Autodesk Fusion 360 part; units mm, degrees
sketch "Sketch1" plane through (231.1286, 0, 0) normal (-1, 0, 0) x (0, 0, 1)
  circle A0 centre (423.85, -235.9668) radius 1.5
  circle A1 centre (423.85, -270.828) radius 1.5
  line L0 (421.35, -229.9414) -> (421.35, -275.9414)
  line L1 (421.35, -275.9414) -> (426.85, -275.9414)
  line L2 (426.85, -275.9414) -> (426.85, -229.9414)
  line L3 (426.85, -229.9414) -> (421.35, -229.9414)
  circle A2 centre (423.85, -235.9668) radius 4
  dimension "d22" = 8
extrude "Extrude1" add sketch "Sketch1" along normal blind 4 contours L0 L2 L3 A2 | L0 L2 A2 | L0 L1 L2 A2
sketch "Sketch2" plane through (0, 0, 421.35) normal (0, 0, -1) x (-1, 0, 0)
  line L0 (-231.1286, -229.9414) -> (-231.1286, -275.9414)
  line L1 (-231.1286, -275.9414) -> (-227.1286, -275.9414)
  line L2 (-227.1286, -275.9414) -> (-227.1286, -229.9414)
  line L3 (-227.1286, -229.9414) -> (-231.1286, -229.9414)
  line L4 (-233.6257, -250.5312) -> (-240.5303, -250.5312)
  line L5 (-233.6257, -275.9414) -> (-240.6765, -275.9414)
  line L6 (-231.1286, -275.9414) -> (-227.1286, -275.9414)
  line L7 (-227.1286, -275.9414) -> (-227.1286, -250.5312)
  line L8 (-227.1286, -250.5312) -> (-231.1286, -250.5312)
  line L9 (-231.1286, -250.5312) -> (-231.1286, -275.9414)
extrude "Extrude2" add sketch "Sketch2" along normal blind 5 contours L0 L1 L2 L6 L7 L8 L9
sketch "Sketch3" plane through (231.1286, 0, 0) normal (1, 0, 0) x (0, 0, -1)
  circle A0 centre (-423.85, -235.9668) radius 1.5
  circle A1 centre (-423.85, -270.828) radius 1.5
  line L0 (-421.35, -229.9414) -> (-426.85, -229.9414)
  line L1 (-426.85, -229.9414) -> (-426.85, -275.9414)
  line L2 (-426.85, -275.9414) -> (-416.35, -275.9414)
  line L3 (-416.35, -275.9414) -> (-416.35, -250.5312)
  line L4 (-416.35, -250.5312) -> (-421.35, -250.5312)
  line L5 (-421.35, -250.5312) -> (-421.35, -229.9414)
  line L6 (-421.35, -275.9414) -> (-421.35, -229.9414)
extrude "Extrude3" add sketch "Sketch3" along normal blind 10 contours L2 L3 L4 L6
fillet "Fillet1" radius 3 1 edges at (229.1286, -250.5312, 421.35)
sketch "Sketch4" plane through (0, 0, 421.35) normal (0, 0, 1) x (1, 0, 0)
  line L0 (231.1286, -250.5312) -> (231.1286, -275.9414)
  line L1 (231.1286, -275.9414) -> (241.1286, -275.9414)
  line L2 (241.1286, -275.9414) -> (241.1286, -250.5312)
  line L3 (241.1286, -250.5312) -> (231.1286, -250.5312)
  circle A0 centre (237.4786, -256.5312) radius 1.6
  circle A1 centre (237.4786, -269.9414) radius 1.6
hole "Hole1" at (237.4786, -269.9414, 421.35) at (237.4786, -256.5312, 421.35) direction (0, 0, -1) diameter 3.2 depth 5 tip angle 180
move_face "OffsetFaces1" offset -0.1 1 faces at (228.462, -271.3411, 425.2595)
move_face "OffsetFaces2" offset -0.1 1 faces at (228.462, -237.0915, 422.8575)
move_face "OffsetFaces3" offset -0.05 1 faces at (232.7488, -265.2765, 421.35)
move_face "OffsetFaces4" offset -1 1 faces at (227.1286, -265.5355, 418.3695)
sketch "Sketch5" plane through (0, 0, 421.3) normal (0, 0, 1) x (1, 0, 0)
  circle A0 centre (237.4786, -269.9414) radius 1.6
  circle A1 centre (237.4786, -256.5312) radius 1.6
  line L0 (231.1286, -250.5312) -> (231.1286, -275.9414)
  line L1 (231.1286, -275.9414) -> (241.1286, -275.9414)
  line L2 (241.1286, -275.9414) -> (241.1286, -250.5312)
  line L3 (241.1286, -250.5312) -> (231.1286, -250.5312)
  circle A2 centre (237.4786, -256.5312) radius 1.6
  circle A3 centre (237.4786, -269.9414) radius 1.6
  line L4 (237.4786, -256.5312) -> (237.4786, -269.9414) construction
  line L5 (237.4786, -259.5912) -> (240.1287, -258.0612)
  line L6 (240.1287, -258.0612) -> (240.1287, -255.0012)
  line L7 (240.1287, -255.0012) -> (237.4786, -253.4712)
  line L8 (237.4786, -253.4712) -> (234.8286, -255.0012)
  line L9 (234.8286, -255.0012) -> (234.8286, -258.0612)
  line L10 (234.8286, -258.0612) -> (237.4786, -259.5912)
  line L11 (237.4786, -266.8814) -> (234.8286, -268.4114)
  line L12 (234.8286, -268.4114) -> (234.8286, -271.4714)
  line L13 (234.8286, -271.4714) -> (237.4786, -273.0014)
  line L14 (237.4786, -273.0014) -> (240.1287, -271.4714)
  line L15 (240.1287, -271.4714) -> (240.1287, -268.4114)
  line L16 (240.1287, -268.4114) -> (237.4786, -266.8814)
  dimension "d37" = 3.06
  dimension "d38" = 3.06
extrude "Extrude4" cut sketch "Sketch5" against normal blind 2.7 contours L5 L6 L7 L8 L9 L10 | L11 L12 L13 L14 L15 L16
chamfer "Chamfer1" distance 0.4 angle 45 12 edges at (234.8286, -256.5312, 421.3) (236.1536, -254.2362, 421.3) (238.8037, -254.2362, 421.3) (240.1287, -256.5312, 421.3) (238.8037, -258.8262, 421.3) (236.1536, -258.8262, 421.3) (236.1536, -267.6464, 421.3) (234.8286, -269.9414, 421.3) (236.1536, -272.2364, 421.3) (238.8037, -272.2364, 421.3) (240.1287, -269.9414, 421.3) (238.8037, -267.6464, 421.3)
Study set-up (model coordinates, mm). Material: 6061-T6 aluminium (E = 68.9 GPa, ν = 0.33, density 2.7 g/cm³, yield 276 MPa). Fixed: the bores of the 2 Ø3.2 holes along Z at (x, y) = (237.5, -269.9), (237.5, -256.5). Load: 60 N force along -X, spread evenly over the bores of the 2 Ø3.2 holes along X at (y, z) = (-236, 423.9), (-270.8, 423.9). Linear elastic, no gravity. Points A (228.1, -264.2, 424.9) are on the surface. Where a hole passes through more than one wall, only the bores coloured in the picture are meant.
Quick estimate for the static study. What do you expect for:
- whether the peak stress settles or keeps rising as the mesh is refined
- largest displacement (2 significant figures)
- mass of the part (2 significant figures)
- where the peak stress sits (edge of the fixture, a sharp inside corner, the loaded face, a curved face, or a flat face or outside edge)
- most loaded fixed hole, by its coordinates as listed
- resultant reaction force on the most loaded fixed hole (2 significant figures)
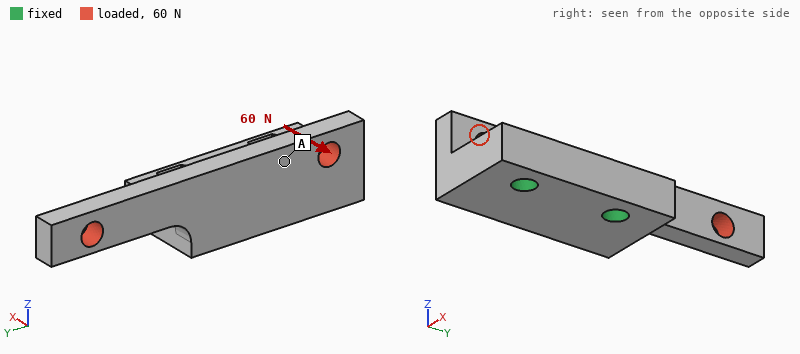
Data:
keeps rising
99 µm
5.9 g
a sharp inside corner
(237.5, -256.5)
69 N
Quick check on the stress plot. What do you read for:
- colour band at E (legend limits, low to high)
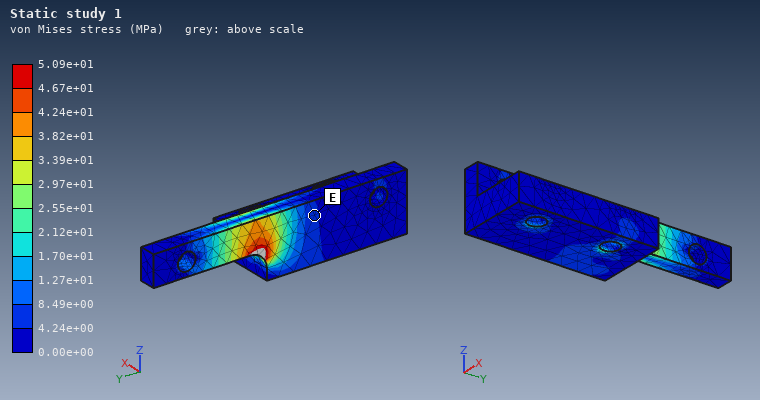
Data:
4.24e+00 to 8.49e+00 MPa
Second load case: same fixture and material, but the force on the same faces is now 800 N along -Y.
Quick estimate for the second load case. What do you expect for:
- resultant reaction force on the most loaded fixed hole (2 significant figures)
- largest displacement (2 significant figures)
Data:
660 N
41 µm
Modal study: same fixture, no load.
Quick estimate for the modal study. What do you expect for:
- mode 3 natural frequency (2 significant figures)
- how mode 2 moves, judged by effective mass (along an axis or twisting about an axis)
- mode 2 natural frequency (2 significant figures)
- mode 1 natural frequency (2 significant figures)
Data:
13 kHz
along Z
7300 Hz
4500 Hz
